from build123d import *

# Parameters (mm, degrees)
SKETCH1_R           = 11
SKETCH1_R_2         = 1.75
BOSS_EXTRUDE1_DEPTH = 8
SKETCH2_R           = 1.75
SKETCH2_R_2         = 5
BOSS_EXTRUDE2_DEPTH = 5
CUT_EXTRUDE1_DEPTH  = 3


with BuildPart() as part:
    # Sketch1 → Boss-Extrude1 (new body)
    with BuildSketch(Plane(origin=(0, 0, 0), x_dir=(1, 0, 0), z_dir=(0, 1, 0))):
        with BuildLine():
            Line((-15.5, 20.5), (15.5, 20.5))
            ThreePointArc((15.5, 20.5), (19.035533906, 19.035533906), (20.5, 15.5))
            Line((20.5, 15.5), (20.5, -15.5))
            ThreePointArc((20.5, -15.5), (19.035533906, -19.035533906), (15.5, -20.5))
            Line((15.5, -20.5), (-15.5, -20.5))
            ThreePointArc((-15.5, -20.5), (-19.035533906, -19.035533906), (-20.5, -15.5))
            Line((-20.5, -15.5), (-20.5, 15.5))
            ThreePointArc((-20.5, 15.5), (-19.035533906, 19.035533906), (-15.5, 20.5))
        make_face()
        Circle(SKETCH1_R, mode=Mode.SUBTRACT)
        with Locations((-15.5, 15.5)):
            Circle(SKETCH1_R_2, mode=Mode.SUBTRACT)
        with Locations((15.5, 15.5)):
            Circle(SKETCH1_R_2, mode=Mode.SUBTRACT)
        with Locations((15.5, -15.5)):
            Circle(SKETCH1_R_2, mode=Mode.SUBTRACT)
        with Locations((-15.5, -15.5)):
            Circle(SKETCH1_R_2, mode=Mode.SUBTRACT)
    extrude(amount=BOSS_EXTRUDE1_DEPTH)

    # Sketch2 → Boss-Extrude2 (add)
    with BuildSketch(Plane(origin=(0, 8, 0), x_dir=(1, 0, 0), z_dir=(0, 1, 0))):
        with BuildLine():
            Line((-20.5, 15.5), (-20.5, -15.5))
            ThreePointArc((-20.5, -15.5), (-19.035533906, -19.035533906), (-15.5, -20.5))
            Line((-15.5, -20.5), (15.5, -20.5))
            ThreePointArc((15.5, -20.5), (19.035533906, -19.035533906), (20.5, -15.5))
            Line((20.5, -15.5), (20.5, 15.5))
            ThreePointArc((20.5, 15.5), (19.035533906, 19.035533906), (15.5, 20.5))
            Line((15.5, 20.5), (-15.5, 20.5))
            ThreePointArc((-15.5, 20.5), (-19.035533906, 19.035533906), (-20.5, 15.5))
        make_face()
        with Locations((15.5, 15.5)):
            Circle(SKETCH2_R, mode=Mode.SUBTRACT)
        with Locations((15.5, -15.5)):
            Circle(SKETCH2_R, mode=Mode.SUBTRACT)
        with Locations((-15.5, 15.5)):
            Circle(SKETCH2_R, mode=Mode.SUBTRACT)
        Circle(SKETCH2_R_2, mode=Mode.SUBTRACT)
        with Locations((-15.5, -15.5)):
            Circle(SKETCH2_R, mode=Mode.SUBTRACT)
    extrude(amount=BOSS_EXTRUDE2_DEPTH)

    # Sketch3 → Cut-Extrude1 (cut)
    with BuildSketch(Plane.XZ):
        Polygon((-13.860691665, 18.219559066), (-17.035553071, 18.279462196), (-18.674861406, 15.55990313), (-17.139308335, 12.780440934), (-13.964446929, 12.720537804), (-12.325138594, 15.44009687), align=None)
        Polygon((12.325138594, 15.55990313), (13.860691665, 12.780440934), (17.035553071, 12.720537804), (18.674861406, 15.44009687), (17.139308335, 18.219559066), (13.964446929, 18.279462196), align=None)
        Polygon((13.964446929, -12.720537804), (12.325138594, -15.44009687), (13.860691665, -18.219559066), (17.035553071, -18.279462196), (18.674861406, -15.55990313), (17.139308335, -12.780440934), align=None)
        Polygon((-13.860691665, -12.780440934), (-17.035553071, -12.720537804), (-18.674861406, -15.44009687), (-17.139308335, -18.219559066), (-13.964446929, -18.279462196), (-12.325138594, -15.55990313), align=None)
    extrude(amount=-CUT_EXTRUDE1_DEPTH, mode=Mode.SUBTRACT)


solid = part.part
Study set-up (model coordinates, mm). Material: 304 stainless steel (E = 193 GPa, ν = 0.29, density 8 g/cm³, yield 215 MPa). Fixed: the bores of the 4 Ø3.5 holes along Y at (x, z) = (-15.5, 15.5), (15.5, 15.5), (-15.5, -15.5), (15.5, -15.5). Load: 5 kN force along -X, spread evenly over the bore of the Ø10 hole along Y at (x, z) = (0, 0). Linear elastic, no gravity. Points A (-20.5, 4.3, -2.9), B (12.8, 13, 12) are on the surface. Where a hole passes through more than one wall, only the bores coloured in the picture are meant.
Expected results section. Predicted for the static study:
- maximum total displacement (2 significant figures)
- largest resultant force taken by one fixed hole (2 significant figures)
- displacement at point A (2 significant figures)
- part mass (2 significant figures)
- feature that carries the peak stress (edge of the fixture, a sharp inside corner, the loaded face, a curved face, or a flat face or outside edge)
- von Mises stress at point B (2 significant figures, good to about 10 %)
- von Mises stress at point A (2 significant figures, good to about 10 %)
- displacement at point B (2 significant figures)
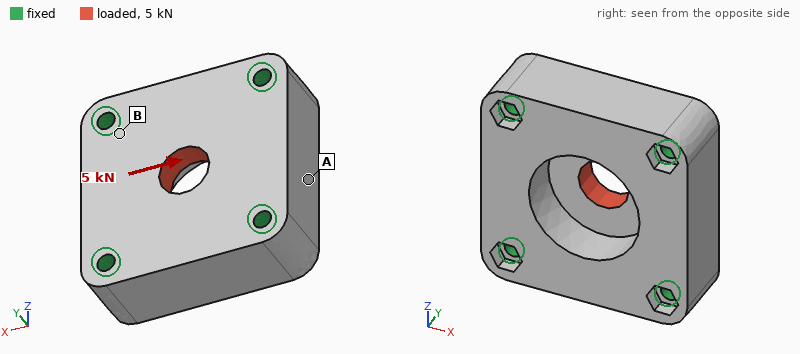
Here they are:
2.6 µm
1.4 kN
0.91 µm
140 g
the loaded face
23 MPa
8.4 MPa
0.48 µm
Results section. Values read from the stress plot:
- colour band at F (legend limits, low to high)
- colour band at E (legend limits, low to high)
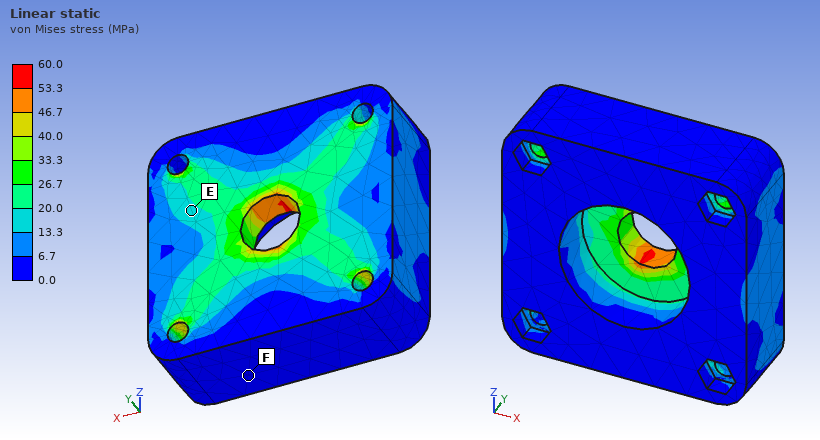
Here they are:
0.0 to 6.7 MPa
13.3 to 20.0 MPa
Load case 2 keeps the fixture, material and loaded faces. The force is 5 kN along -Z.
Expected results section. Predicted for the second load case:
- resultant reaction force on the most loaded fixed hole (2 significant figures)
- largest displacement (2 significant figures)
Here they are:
1.4 kN
2.6 µm
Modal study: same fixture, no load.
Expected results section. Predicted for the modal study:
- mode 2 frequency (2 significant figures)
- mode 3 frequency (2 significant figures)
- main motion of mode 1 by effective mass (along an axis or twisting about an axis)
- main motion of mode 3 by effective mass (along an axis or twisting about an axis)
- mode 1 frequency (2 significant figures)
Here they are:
32 kHz
36 kHz
along Y
twisting about X
28 kHz
